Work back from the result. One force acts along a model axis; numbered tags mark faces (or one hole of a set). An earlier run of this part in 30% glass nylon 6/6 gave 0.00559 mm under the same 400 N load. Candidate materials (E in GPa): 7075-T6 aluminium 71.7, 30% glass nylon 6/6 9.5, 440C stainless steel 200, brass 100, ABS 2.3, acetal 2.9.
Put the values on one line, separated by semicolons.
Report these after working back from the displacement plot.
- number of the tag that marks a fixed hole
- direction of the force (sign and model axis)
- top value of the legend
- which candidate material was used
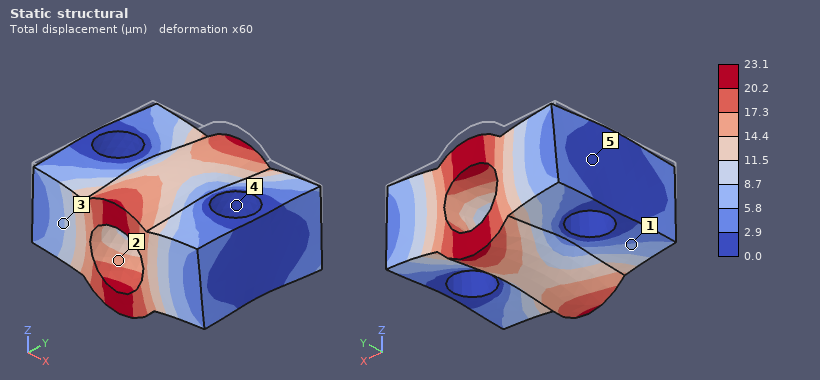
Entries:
4; -Z; 23.1 µm; ABS
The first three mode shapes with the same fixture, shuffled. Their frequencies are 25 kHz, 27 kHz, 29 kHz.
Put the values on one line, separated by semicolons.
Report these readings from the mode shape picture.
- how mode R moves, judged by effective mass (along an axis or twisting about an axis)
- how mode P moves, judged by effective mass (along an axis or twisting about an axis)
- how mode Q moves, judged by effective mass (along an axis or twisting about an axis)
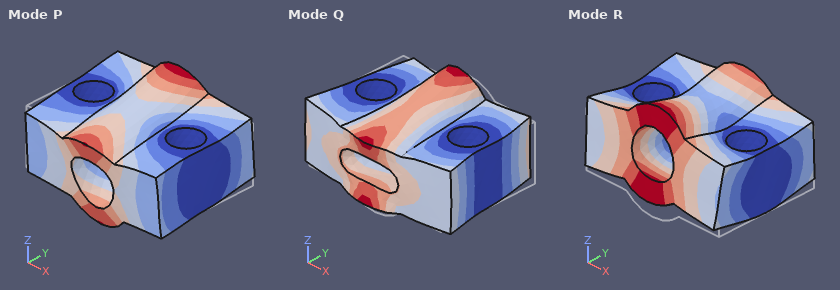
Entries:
along Z; twisting about X; along Y
